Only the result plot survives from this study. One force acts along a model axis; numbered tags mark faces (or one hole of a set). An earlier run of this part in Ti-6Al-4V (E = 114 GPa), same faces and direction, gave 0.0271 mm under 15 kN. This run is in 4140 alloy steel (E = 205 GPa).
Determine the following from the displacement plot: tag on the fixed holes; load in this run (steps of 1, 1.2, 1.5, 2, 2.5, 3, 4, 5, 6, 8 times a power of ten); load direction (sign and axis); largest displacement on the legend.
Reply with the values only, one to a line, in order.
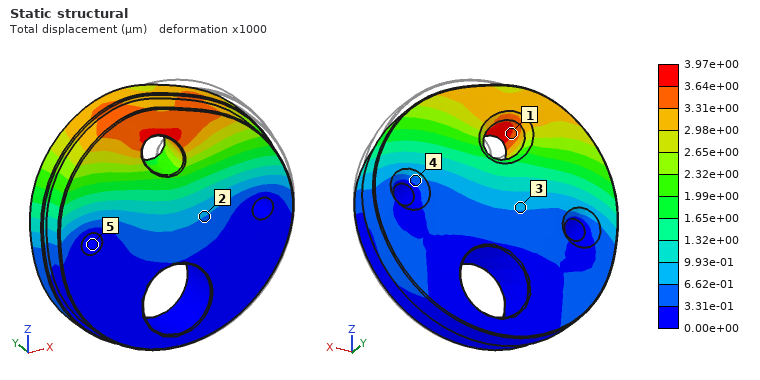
5
4 kN
-X
3.97e+00 µm
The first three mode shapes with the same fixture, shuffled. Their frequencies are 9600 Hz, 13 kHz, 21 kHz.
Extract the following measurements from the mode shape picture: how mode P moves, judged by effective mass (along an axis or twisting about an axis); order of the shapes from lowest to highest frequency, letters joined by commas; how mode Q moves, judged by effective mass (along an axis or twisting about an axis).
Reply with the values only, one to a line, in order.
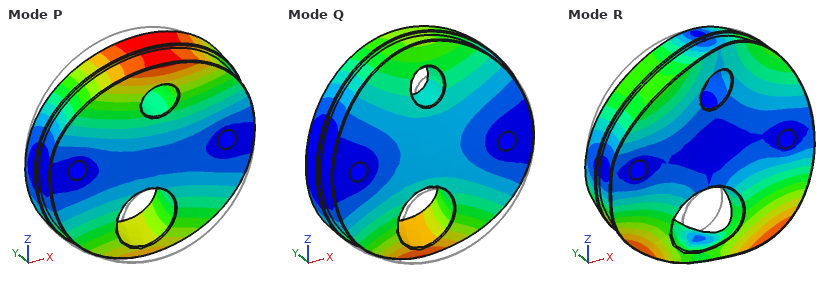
twisting about X
P, Q, R
along Y
